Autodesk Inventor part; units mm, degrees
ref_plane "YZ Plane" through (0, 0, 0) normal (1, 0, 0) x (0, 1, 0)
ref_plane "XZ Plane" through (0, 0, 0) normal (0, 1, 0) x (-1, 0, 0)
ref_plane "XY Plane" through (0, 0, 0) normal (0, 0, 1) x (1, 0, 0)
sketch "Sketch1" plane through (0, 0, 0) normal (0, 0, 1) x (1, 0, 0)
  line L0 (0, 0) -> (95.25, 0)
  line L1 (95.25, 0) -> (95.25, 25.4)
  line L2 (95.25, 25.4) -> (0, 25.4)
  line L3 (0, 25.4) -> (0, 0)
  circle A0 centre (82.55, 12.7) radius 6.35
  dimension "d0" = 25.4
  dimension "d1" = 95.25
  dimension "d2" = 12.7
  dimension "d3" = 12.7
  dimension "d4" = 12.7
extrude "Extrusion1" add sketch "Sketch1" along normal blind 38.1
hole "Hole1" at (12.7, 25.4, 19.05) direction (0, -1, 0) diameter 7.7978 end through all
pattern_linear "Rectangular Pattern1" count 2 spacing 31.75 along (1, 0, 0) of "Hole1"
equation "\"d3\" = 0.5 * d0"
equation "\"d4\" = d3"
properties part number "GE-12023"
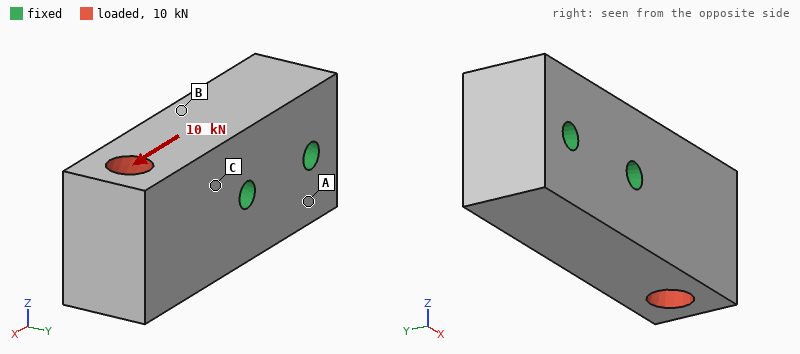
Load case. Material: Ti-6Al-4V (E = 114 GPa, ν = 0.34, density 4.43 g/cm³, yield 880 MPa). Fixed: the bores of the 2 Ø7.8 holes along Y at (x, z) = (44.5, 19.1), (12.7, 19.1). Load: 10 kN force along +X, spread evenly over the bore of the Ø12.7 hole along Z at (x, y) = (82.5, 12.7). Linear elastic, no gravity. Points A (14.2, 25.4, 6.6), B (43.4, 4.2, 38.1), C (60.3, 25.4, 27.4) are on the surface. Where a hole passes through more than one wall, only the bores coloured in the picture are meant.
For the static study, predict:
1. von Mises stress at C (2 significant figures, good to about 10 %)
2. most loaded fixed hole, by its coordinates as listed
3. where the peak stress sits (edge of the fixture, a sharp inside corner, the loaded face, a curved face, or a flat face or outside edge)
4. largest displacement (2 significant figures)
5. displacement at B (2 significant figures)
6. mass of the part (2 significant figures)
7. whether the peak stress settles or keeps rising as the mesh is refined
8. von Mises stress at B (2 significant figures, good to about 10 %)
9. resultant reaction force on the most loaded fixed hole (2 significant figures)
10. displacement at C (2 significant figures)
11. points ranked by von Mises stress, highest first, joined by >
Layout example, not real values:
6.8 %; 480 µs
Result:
12 MPa; (44.5, 19.1); edge of the fixture; 6.4 µm; 1.3 µm; 380 g; keeps rising; 6.1 MPa; 8.2 kN; 2.1 µm; C > B > A
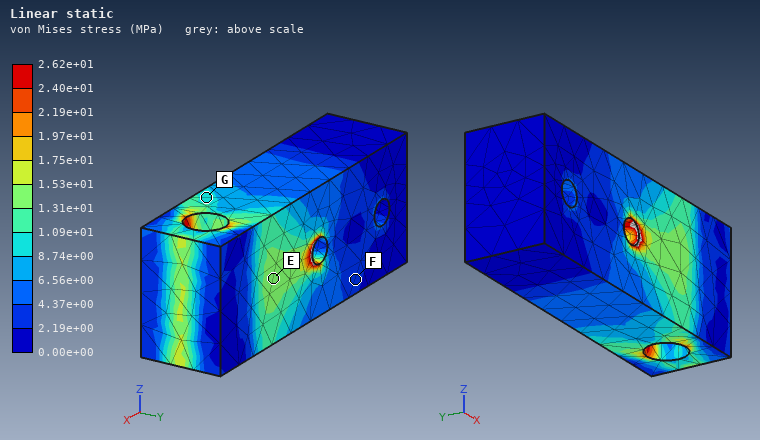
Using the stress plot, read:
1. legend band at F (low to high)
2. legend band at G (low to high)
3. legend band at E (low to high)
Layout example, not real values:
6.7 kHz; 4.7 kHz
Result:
2.19e+00 to 4.37e+00 MPa; 8.74e+00 to 1.09e+01 MPa; 1.31e+01 to 1.53e+01 MPa
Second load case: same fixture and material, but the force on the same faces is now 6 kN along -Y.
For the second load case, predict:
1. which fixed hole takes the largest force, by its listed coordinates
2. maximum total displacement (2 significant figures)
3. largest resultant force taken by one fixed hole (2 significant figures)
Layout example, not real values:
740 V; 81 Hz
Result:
(44.5, 19.1); 45 µm; 7.6 kN
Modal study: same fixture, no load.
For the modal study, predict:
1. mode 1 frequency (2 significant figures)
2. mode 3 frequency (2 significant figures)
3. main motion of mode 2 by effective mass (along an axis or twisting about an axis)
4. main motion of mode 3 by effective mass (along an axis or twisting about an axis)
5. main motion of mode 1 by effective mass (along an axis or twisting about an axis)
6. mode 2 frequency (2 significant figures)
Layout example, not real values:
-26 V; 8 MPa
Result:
6700 Hz; 13 kHz; along Z; twisting about X; along Y; 7200 Hz
